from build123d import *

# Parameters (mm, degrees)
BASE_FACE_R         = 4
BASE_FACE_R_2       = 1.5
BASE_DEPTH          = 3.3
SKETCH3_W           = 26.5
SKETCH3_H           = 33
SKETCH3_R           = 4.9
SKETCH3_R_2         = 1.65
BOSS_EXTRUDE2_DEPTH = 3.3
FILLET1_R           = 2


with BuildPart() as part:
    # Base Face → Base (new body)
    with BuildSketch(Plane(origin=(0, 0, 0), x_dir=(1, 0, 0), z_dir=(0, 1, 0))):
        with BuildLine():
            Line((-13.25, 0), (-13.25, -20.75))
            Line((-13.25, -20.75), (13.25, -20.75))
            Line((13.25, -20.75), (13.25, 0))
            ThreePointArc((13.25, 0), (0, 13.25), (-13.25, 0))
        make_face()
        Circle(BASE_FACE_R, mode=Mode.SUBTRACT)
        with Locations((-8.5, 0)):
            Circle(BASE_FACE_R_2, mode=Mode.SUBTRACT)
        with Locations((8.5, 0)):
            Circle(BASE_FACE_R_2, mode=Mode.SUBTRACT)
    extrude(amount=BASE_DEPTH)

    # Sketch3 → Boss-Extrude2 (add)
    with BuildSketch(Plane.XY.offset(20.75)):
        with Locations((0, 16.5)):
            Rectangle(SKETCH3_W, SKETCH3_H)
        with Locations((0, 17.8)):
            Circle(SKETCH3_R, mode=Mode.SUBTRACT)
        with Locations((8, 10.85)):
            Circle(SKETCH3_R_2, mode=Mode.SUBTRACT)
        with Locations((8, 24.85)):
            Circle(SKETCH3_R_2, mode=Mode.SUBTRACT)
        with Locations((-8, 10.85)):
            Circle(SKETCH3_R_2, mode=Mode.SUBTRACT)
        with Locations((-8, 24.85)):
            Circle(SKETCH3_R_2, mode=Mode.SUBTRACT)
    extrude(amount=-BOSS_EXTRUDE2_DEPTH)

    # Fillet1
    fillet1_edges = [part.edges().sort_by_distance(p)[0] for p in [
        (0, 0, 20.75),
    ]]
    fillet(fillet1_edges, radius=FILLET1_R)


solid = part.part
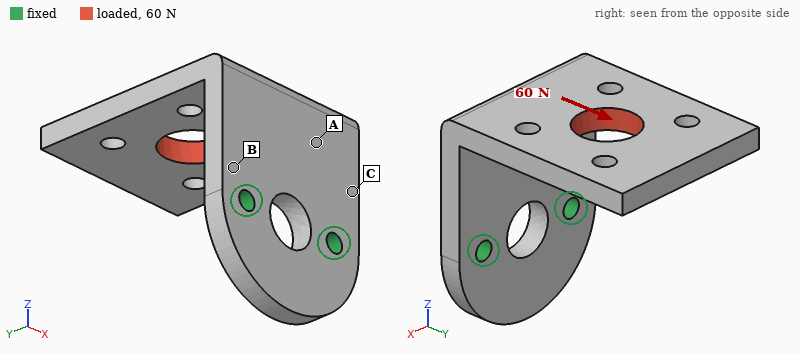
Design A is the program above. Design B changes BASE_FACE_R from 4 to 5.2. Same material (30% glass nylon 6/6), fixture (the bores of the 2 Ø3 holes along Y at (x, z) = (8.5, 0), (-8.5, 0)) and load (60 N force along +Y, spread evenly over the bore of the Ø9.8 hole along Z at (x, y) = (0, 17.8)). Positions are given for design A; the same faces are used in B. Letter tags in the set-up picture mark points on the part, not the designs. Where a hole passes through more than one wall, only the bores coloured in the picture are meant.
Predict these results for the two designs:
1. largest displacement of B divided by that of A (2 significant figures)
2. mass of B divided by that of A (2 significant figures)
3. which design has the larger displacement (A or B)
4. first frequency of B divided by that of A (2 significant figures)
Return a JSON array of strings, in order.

["1.1", "0.98", "B", "0.97"]
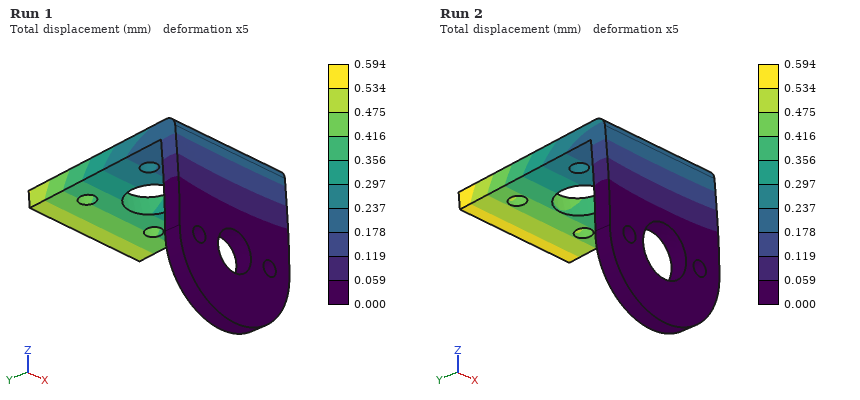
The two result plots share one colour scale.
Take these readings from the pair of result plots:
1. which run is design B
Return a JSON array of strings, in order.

["Run 2"]
